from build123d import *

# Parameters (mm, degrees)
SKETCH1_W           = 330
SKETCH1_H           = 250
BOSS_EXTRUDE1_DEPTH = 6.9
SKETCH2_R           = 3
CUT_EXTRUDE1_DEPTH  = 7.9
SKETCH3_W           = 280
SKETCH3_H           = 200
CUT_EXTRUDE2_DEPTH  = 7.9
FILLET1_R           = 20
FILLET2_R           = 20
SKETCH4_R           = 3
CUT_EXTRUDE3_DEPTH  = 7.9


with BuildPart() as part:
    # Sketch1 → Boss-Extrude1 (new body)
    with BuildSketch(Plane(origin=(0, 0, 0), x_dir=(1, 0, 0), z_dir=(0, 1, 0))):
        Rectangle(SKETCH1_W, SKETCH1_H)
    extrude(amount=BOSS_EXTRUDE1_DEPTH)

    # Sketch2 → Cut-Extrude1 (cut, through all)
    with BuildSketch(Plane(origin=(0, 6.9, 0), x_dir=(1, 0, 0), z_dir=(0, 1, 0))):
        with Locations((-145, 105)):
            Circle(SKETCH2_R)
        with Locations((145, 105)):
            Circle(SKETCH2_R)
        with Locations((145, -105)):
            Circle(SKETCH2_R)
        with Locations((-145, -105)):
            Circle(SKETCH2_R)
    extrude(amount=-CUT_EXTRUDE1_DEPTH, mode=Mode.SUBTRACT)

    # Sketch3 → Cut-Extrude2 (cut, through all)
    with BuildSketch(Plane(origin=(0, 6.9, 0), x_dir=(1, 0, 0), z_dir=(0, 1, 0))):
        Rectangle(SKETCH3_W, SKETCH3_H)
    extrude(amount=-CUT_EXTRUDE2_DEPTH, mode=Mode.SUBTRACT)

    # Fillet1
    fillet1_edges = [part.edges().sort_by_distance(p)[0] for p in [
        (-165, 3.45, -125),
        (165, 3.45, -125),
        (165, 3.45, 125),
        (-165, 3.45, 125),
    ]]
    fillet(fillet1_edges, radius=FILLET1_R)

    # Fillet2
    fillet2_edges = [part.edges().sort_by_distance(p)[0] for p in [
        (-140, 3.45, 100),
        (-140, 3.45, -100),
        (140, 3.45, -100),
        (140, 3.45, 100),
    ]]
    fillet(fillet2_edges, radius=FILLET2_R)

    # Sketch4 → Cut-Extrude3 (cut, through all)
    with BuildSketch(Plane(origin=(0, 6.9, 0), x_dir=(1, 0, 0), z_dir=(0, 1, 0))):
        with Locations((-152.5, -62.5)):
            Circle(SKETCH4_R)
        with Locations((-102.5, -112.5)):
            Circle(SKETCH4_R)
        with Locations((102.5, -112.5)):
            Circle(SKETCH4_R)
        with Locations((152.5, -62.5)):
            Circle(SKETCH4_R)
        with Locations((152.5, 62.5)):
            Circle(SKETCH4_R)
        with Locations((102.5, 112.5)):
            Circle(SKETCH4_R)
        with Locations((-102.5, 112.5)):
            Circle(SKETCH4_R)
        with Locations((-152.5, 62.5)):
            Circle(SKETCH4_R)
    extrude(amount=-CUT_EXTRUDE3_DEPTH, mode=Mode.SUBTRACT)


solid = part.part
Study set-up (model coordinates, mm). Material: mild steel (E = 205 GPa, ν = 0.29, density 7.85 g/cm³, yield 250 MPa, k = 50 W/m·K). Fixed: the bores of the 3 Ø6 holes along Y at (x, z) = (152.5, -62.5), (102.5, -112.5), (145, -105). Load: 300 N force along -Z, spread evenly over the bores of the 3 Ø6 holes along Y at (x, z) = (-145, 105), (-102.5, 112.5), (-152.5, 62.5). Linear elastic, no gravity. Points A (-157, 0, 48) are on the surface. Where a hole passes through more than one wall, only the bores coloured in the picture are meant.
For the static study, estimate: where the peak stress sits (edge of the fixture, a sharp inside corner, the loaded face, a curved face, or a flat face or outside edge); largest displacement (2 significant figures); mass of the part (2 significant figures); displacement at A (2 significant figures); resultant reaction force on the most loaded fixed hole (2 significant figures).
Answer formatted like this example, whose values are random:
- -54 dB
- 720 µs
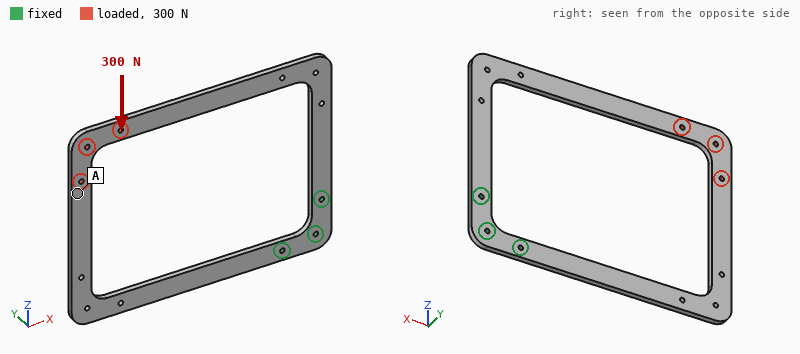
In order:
- edge of the fixture
- 0.44 mm
- 1.4 kg
- 0.42 mm
- 860 N
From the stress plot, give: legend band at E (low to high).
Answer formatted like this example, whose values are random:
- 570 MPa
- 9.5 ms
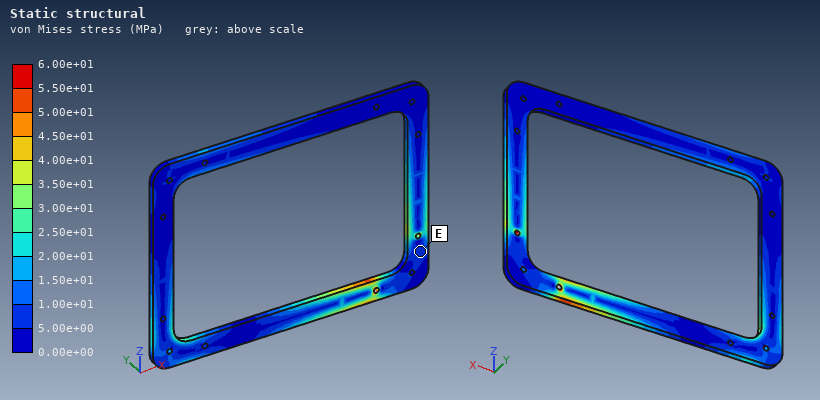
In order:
- 5.00e+00 to 1.00e+01 MPa
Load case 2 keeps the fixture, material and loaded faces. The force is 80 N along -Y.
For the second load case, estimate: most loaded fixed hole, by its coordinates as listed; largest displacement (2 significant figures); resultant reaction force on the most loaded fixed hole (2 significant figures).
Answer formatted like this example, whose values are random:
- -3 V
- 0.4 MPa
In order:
- (102.5, -112.5)
- 4.5 mm
- 84 N
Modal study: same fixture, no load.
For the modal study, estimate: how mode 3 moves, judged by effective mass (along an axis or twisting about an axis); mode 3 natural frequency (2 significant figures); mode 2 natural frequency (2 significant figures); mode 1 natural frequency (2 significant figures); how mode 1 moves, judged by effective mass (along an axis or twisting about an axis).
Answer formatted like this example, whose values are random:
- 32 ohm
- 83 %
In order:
- along Y
- 160 Hz
- 81 Hz
- 35 Hz
- along Y
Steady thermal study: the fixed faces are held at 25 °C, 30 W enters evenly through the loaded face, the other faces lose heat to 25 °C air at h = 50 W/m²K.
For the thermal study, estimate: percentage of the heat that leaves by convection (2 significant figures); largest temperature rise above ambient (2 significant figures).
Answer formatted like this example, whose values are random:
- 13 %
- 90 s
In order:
- 100 %
- 55 K
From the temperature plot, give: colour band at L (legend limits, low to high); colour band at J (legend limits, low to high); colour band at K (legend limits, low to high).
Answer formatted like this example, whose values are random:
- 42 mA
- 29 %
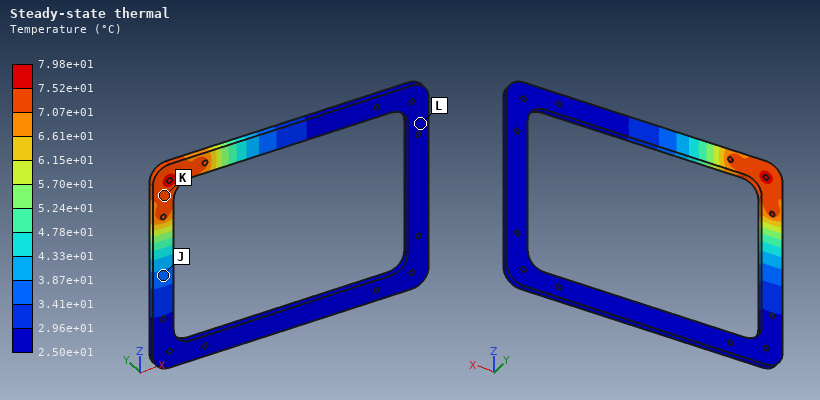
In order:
- 2.50e+01 to 2.96e+01 °C
- 3.41e+01 to 3.87e+01 °C
- 7.07e+01 to 7.52e+01 °C
